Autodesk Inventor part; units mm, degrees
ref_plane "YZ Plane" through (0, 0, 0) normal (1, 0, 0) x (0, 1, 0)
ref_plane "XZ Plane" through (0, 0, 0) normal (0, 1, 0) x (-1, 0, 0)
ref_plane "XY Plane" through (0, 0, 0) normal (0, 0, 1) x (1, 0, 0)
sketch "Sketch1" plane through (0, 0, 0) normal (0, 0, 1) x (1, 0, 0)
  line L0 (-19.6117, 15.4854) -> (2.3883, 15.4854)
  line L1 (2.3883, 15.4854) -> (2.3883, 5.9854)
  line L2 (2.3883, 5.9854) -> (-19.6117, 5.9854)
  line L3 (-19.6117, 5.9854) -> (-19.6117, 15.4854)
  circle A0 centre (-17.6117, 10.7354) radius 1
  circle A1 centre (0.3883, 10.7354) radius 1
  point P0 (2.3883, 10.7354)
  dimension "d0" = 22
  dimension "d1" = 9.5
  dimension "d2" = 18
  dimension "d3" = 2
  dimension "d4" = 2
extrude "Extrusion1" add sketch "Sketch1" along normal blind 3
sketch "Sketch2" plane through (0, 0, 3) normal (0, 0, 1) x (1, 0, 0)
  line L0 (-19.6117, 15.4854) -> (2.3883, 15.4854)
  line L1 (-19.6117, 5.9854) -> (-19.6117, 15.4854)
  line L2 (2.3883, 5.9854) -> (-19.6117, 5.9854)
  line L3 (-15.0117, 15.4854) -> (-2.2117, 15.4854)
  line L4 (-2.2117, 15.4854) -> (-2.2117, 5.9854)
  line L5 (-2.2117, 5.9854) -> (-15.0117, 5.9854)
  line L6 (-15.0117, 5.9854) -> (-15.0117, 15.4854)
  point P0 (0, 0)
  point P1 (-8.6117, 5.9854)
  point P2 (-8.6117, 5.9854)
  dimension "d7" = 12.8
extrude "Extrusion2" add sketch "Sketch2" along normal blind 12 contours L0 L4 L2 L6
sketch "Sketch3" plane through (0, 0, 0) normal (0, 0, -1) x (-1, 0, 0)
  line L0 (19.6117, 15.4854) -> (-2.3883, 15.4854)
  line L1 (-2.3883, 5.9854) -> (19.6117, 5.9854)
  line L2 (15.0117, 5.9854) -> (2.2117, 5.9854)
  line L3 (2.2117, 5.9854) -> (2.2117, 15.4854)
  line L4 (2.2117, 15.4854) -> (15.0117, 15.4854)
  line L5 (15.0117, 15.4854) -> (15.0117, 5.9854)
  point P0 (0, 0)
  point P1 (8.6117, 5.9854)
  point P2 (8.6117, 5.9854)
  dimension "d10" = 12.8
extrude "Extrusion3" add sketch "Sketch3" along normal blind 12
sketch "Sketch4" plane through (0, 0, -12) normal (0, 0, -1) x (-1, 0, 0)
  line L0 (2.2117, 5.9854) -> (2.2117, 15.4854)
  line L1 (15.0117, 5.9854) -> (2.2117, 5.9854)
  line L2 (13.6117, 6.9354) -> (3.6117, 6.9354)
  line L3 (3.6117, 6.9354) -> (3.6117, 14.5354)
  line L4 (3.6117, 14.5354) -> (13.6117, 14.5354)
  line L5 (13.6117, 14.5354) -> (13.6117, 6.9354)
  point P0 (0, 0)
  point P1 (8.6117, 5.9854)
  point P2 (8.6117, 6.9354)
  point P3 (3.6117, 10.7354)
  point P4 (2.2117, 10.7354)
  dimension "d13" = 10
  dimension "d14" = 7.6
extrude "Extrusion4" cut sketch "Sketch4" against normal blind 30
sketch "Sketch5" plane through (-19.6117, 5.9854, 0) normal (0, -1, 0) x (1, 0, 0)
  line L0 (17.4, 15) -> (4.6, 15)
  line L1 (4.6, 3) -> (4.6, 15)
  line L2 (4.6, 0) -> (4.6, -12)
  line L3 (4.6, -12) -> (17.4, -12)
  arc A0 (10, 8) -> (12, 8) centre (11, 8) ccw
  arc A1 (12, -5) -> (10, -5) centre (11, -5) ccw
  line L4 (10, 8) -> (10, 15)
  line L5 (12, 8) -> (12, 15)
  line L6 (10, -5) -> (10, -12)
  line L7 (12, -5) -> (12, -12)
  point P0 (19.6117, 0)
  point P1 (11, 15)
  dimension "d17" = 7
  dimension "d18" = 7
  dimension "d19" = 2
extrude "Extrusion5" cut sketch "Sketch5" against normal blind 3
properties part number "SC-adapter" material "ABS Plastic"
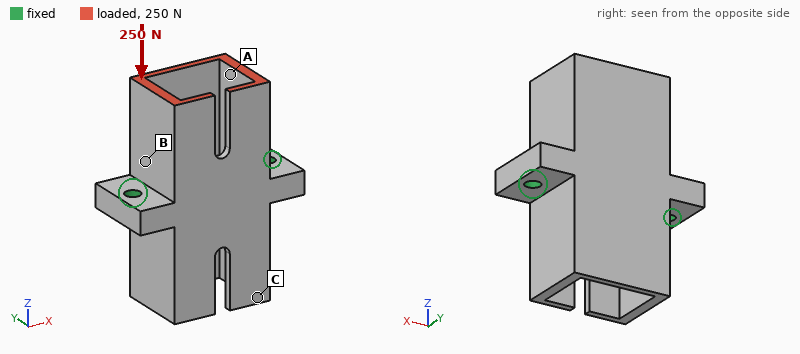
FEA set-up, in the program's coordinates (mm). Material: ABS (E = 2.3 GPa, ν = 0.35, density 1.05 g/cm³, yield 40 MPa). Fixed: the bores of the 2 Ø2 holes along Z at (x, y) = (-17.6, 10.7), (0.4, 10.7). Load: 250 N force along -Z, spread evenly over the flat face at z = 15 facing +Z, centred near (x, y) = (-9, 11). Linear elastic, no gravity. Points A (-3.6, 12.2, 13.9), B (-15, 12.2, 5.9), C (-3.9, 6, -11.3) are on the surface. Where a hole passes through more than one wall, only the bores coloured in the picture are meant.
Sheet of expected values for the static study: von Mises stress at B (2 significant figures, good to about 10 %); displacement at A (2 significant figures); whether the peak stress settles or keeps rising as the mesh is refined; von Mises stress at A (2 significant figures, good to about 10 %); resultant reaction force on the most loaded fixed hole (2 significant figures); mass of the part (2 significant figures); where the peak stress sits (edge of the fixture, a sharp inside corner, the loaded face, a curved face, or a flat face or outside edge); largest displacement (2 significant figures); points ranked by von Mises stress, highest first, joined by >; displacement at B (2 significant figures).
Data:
8.6 MPa
77 µm
keeps rising
6.2 MPa
130 N
1.5 g
edge of the fixture
89 µm
B > A > C
55 µm
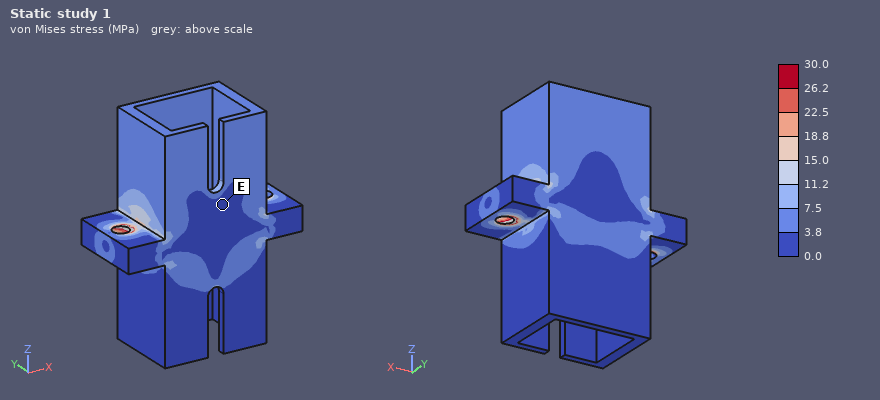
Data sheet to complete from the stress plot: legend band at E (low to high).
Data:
0.0 to 3.8 MPa
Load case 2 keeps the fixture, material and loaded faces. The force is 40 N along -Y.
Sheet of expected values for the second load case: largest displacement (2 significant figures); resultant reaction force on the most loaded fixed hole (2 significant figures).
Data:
0.37 mm
20 N
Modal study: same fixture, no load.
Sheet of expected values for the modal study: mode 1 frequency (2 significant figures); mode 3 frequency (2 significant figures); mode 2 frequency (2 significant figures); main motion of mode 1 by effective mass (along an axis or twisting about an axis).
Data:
3100 Hz
6400 Hz
4900 Hz
twisting about X
